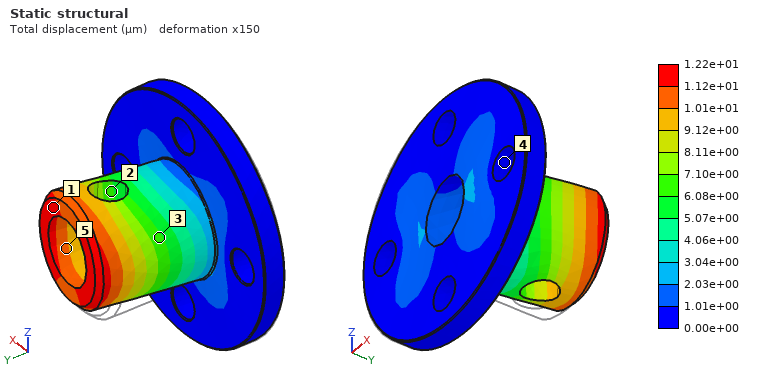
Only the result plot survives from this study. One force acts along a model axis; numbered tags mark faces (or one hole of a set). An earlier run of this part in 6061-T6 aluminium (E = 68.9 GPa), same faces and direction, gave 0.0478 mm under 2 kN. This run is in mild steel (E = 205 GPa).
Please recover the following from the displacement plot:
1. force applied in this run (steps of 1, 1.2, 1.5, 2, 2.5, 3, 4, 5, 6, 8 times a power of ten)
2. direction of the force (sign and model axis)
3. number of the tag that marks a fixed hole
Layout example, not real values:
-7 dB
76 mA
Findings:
1.5 kN
+X
4
